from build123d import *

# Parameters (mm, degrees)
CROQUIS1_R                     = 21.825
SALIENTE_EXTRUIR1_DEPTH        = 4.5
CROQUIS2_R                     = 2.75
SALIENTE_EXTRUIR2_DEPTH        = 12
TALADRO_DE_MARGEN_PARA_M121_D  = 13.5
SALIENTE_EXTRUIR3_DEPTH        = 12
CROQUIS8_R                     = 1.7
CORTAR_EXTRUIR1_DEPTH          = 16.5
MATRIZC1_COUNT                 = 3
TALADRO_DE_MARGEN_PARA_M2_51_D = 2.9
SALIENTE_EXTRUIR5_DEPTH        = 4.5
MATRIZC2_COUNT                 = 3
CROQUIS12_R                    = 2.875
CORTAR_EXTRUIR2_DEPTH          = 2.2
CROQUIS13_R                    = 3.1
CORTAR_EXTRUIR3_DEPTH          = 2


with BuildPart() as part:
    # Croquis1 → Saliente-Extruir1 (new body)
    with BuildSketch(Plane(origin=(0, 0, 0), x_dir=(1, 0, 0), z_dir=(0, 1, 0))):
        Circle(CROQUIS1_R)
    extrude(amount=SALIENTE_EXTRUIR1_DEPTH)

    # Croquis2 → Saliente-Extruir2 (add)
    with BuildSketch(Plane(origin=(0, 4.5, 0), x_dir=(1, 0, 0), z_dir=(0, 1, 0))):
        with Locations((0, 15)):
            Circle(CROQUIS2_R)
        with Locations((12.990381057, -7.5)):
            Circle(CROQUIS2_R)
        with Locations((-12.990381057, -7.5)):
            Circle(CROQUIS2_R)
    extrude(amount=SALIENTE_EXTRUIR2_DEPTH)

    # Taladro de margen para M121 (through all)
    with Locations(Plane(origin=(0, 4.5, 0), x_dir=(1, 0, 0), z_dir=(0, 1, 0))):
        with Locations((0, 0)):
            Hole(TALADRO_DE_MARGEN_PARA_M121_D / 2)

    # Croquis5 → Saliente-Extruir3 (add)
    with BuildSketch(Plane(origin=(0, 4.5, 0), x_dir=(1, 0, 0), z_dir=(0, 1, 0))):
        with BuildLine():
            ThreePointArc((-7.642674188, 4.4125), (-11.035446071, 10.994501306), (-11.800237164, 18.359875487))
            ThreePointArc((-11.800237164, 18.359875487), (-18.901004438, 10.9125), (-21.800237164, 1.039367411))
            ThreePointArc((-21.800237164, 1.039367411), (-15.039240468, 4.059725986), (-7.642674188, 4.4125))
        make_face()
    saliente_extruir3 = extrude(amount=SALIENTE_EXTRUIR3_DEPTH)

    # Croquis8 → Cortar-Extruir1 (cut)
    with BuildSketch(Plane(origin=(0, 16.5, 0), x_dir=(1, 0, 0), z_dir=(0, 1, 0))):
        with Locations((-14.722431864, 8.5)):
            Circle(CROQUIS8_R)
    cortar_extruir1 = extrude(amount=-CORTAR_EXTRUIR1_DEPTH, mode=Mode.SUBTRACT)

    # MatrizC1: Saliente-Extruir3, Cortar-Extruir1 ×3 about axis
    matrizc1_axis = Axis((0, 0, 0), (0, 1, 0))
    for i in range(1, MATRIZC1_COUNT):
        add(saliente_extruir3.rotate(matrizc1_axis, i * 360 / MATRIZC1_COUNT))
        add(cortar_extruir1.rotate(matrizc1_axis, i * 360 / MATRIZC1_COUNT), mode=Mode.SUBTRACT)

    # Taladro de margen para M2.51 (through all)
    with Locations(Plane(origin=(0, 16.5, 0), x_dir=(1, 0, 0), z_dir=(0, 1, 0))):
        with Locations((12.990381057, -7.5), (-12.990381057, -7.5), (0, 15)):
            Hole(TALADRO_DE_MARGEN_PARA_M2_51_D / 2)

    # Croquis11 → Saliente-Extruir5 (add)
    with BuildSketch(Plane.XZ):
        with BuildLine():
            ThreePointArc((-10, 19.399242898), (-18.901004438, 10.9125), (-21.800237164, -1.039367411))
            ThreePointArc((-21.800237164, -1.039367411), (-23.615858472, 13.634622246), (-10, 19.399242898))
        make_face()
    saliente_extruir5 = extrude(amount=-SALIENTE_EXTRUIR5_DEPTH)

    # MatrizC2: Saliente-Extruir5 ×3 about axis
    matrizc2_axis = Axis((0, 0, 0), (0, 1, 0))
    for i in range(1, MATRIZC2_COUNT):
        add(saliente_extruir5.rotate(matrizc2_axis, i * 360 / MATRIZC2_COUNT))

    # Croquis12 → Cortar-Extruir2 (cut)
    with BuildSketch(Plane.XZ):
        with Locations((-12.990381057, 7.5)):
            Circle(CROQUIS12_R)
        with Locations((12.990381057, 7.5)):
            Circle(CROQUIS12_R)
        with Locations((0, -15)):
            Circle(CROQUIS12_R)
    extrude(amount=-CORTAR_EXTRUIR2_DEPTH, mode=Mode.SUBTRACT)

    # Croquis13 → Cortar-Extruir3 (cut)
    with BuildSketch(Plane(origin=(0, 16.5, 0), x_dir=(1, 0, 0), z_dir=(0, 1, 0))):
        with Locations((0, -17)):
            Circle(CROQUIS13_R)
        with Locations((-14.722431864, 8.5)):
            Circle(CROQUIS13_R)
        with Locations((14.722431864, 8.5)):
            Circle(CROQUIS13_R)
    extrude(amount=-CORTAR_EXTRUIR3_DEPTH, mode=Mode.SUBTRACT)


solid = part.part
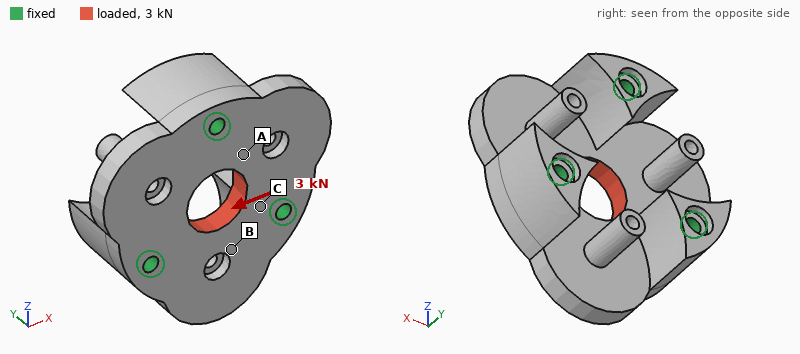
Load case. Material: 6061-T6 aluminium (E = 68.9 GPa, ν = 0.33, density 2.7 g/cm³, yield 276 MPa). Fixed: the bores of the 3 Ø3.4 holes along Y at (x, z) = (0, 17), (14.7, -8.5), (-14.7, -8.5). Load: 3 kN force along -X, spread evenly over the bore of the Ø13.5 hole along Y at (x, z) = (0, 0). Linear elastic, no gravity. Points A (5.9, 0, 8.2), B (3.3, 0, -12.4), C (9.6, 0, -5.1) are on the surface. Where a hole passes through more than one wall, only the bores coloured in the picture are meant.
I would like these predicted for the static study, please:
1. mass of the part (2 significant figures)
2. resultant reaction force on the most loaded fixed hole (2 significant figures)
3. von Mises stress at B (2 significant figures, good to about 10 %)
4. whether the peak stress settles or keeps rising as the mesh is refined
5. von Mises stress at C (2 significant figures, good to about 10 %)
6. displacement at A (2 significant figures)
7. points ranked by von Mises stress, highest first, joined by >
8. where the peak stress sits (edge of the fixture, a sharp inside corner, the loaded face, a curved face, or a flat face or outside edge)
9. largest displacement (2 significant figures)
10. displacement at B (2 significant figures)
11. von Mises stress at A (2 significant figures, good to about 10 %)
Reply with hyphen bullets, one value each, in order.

- 30 g
- 1.0 kN
- 5.3 MPa
- keeps rising
- 19 MPa
- 4.1 µm
- C > A > B
- edge of the fixture
- 5.5 µm
- 1.3 µm
- 13 MPa
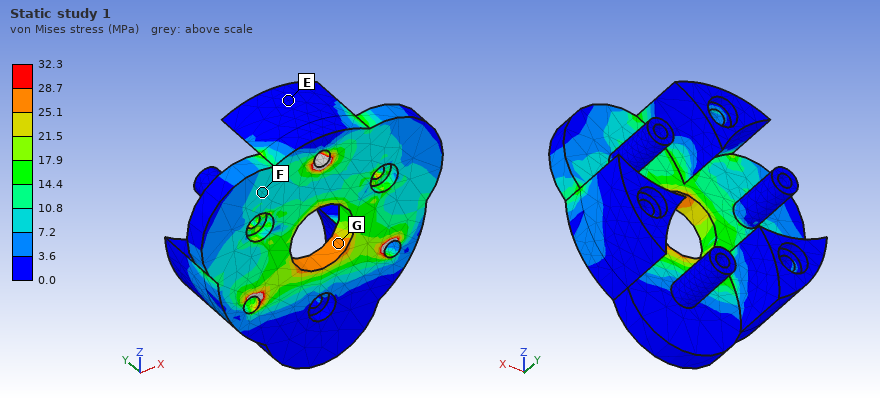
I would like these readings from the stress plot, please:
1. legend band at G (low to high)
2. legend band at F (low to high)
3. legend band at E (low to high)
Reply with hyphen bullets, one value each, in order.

- 25.1 to 28.7 MPa
- 7.2 to 10.8 MPa
- 0.0 to 3.6 MPa
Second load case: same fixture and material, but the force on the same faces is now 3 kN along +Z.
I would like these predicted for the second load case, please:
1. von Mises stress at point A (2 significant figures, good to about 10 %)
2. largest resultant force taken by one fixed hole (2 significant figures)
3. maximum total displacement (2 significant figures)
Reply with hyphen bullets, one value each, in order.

- 15 MPa
- 1.0 kN
- 6.1 µm
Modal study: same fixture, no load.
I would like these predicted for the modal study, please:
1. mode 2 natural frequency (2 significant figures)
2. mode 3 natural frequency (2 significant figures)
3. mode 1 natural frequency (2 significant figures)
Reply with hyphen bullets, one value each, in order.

- 14 kHz
- 14 kHz
- 14 kHz
